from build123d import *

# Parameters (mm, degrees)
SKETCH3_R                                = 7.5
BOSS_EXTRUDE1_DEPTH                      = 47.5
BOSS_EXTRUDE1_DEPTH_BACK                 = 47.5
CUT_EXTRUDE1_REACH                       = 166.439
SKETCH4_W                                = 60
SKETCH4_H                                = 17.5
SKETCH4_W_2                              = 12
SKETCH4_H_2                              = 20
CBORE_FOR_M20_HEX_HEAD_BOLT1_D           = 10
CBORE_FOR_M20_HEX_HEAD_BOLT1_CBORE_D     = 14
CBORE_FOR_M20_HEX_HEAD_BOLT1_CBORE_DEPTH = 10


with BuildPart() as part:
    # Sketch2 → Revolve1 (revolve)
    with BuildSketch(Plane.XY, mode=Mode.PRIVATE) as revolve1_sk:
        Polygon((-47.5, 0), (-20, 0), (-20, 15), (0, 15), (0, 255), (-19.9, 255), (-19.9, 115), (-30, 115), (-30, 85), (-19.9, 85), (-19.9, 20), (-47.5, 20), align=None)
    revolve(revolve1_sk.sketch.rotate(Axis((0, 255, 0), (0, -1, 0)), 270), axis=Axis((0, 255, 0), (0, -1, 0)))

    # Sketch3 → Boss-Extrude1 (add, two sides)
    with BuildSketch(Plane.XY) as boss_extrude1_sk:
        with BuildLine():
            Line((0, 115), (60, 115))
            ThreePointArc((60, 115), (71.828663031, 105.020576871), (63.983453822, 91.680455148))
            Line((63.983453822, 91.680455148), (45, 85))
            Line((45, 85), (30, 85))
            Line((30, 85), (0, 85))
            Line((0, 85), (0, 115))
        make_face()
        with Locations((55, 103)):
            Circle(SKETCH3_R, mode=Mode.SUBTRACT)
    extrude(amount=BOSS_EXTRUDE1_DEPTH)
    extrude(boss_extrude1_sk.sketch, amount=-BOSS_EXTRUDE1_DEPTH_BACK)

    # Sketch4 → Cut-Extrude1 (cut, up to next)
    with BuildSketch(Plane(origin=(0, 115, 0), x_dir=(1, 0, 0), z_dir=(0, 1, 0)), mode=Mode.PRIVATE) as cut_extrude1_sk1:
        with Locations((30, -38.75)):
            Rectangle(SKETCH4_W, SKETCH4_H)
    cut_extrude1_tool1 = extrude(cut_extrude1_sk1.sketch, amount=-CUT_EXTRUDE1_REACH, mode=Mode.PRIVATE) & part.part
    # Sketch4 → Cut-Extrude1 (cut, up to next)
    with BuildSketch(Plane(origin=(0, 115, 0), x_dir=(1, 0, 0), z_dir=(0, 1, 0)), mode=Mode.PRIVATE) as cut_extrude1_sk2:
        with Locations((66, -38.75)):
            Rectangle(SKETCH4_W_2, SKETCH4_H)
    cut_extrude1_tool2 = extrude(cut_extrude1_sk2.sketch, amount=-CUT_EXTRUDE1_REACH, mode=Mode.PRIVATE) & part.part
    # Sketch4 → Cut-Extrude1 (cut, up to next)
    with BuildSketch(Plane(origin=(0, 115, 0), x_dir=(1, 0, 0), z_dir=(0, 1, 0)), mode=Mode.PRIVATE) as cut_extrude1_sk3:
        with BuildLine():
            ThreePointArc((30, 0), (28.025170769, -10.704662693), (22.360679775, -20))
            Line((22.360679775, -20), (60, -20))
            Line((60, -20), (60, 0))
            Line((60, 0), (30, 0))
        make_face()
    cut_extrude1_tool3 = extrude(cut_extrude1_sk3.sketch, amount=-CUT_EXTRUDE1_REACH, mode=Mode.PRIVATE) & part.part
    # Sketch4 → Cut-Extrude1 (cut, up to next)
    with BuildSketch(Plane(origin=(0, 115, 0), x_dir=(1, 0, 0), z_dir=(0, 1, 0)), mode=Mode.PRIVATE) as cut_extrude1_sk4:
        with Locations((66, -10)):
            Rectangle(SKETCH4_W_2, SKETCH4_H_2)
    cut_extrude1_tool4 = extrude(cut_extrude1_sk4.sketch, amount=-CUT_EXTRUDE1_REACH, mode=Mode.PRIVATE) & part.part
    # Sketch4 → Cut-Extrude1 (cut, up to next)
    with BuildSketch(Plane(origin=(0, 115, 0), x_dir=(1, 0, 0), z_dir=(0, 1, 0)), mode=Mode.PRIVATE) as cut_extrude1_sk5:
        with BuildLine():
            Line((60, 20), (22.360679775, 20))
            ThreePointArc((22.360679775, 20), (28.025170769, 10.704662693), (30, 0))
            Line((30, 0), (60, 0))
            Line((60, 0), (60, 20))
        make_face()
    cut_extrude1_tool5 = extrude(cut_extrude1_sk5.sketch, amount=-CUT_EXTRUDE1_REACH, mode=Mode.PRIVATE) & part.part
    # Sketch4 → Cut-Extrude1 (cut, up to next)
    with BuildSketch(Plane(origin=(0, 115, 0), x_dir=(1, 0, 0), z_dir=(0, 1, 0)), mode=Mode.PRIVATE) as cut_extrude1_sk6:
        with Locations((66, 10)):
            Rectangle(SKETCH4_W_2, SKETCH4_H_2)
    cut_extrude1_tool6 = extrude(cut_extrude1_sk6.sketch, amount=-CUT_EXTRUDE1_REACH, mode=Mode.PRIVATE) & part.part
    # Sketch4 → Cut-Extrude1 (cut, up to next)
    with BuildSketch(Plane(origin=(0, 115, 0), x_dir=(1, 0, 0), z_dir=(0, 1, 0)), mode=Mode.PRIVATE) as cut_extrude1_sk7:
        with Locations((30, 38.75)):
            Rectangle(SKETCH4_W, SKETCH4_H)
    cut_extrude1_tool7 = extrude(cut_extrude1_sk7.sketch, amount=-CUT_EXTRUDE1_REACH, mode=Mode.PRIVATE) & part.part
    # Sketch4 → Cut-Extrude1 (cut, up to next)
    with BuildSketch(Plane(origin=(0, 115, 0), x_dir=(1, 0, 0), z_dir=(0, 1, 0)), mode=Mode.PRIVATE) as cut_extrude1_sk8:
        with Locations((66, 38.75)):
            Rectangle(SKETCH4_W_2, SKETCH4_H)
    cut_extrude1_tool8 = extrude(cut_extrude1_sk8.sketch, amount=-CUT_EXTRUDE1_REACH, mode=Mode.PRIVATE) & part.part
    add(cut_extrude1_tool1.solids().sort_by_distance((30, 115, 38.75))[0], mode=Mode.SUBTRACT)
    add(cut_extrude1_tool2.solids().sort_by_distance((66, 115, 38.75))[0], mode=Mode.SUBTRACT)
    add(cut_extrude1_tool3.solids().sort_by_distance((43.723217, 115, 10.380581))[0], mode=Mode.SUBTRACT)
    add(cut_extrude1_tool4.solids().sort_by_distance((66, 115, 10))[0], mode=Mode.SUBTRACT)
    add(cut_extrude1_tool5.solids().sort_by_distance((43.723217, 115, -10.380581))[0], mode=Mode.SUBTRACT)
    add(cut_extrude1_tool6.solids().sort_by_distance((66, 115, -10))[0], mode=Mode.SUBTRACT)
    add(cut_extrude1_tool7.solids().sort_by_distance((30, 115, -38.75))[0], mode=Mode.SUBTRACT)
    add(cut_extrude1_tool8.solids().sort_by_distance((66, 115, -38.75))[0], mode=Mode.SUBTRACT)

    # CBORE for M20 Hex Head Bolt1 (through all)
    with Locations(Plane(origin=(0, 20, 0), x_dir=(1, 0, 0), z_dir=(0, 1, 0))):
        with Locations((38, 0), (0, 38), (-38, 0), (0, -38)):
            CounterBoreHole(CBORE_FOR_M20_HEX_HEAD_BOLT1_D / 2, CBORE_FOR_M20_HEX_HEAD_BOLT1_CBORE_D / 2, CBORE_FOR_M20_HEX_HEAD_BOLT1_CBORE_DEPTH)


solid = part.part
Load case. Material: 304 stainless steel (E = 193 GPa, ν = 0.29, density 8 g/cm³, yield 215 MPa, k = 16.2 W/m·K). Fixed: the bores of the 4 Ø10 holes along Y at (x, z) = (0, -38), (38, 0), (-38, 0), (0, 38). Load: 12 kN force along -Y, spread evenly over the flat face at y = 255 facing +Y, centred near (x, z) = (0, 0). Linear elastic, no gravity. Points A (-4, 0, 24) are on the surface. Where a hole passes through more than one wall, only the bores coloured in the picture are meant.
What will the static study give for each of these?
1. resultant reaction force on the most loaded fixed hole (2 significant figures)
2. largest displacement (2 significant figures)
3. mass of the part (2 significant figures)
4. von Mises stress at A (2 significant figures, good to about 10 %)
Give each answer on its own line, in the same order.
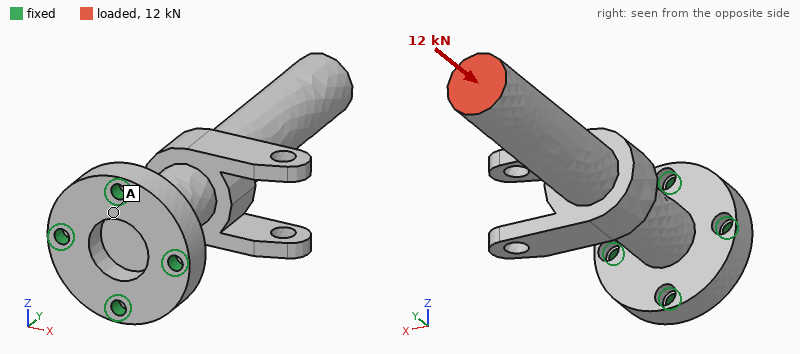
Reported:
3.7 kN
15 µm
3.8 kg
5.6 MPa
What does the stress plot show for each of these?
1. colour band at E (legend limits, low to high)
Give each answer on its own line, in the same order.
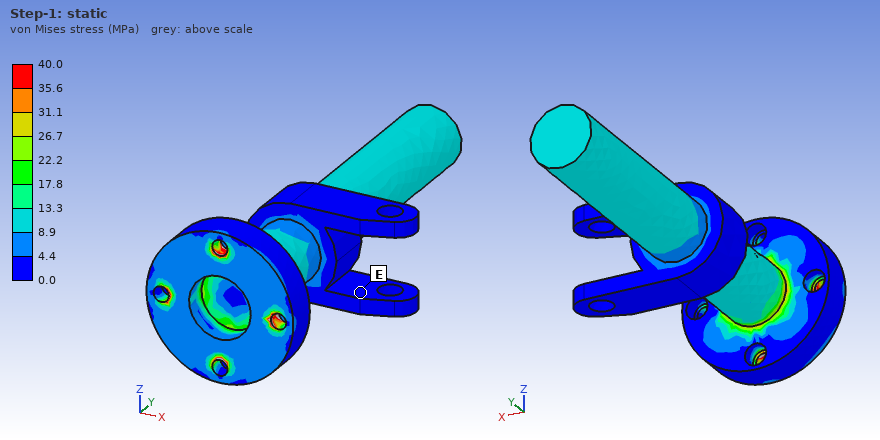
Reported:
0.0 to 4.4 MPa
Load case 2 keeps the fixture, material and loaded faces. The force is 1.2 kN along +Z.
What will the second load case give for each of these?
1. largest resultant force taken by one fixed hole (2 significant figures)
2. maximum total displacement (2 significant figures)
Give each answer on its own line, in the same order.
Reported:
4.7 kN
0.28 mm
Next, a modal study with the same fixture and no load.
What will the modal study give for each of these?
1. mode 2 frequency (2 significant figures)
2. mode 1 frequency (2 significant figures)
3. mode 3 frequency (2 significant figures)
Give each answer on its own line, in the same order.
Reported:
400 Hz
400 Hz
1900 Hz
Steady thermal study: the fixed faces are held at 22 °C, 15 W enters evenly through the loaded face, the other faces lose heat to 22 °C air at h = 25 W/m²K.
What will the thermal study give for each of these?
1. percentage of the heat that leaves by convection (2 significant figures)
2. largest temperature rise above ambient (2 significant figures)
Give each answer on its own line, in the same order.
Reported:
95 %
59 K
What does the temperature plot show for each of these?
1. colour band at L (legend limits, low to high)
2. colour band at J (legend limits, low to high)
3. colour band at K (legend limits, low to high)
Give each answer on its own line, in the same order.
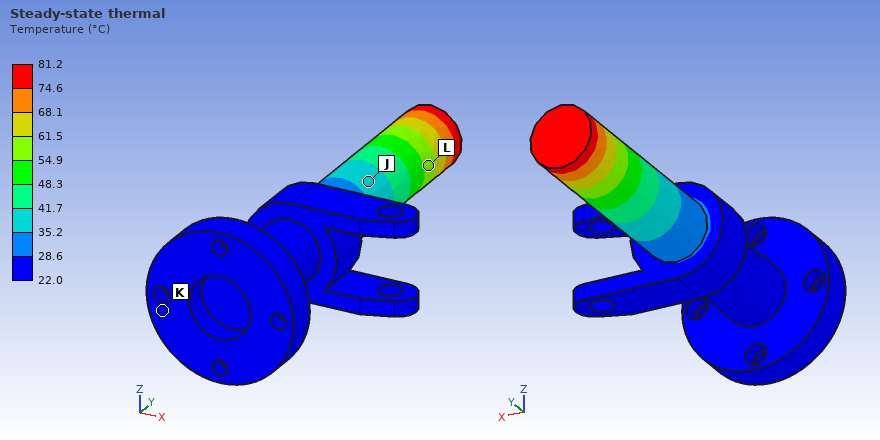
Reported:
54.9 to 61.5 °C
35.2 to 41.7 °C
22.0 to 28.6 °C
